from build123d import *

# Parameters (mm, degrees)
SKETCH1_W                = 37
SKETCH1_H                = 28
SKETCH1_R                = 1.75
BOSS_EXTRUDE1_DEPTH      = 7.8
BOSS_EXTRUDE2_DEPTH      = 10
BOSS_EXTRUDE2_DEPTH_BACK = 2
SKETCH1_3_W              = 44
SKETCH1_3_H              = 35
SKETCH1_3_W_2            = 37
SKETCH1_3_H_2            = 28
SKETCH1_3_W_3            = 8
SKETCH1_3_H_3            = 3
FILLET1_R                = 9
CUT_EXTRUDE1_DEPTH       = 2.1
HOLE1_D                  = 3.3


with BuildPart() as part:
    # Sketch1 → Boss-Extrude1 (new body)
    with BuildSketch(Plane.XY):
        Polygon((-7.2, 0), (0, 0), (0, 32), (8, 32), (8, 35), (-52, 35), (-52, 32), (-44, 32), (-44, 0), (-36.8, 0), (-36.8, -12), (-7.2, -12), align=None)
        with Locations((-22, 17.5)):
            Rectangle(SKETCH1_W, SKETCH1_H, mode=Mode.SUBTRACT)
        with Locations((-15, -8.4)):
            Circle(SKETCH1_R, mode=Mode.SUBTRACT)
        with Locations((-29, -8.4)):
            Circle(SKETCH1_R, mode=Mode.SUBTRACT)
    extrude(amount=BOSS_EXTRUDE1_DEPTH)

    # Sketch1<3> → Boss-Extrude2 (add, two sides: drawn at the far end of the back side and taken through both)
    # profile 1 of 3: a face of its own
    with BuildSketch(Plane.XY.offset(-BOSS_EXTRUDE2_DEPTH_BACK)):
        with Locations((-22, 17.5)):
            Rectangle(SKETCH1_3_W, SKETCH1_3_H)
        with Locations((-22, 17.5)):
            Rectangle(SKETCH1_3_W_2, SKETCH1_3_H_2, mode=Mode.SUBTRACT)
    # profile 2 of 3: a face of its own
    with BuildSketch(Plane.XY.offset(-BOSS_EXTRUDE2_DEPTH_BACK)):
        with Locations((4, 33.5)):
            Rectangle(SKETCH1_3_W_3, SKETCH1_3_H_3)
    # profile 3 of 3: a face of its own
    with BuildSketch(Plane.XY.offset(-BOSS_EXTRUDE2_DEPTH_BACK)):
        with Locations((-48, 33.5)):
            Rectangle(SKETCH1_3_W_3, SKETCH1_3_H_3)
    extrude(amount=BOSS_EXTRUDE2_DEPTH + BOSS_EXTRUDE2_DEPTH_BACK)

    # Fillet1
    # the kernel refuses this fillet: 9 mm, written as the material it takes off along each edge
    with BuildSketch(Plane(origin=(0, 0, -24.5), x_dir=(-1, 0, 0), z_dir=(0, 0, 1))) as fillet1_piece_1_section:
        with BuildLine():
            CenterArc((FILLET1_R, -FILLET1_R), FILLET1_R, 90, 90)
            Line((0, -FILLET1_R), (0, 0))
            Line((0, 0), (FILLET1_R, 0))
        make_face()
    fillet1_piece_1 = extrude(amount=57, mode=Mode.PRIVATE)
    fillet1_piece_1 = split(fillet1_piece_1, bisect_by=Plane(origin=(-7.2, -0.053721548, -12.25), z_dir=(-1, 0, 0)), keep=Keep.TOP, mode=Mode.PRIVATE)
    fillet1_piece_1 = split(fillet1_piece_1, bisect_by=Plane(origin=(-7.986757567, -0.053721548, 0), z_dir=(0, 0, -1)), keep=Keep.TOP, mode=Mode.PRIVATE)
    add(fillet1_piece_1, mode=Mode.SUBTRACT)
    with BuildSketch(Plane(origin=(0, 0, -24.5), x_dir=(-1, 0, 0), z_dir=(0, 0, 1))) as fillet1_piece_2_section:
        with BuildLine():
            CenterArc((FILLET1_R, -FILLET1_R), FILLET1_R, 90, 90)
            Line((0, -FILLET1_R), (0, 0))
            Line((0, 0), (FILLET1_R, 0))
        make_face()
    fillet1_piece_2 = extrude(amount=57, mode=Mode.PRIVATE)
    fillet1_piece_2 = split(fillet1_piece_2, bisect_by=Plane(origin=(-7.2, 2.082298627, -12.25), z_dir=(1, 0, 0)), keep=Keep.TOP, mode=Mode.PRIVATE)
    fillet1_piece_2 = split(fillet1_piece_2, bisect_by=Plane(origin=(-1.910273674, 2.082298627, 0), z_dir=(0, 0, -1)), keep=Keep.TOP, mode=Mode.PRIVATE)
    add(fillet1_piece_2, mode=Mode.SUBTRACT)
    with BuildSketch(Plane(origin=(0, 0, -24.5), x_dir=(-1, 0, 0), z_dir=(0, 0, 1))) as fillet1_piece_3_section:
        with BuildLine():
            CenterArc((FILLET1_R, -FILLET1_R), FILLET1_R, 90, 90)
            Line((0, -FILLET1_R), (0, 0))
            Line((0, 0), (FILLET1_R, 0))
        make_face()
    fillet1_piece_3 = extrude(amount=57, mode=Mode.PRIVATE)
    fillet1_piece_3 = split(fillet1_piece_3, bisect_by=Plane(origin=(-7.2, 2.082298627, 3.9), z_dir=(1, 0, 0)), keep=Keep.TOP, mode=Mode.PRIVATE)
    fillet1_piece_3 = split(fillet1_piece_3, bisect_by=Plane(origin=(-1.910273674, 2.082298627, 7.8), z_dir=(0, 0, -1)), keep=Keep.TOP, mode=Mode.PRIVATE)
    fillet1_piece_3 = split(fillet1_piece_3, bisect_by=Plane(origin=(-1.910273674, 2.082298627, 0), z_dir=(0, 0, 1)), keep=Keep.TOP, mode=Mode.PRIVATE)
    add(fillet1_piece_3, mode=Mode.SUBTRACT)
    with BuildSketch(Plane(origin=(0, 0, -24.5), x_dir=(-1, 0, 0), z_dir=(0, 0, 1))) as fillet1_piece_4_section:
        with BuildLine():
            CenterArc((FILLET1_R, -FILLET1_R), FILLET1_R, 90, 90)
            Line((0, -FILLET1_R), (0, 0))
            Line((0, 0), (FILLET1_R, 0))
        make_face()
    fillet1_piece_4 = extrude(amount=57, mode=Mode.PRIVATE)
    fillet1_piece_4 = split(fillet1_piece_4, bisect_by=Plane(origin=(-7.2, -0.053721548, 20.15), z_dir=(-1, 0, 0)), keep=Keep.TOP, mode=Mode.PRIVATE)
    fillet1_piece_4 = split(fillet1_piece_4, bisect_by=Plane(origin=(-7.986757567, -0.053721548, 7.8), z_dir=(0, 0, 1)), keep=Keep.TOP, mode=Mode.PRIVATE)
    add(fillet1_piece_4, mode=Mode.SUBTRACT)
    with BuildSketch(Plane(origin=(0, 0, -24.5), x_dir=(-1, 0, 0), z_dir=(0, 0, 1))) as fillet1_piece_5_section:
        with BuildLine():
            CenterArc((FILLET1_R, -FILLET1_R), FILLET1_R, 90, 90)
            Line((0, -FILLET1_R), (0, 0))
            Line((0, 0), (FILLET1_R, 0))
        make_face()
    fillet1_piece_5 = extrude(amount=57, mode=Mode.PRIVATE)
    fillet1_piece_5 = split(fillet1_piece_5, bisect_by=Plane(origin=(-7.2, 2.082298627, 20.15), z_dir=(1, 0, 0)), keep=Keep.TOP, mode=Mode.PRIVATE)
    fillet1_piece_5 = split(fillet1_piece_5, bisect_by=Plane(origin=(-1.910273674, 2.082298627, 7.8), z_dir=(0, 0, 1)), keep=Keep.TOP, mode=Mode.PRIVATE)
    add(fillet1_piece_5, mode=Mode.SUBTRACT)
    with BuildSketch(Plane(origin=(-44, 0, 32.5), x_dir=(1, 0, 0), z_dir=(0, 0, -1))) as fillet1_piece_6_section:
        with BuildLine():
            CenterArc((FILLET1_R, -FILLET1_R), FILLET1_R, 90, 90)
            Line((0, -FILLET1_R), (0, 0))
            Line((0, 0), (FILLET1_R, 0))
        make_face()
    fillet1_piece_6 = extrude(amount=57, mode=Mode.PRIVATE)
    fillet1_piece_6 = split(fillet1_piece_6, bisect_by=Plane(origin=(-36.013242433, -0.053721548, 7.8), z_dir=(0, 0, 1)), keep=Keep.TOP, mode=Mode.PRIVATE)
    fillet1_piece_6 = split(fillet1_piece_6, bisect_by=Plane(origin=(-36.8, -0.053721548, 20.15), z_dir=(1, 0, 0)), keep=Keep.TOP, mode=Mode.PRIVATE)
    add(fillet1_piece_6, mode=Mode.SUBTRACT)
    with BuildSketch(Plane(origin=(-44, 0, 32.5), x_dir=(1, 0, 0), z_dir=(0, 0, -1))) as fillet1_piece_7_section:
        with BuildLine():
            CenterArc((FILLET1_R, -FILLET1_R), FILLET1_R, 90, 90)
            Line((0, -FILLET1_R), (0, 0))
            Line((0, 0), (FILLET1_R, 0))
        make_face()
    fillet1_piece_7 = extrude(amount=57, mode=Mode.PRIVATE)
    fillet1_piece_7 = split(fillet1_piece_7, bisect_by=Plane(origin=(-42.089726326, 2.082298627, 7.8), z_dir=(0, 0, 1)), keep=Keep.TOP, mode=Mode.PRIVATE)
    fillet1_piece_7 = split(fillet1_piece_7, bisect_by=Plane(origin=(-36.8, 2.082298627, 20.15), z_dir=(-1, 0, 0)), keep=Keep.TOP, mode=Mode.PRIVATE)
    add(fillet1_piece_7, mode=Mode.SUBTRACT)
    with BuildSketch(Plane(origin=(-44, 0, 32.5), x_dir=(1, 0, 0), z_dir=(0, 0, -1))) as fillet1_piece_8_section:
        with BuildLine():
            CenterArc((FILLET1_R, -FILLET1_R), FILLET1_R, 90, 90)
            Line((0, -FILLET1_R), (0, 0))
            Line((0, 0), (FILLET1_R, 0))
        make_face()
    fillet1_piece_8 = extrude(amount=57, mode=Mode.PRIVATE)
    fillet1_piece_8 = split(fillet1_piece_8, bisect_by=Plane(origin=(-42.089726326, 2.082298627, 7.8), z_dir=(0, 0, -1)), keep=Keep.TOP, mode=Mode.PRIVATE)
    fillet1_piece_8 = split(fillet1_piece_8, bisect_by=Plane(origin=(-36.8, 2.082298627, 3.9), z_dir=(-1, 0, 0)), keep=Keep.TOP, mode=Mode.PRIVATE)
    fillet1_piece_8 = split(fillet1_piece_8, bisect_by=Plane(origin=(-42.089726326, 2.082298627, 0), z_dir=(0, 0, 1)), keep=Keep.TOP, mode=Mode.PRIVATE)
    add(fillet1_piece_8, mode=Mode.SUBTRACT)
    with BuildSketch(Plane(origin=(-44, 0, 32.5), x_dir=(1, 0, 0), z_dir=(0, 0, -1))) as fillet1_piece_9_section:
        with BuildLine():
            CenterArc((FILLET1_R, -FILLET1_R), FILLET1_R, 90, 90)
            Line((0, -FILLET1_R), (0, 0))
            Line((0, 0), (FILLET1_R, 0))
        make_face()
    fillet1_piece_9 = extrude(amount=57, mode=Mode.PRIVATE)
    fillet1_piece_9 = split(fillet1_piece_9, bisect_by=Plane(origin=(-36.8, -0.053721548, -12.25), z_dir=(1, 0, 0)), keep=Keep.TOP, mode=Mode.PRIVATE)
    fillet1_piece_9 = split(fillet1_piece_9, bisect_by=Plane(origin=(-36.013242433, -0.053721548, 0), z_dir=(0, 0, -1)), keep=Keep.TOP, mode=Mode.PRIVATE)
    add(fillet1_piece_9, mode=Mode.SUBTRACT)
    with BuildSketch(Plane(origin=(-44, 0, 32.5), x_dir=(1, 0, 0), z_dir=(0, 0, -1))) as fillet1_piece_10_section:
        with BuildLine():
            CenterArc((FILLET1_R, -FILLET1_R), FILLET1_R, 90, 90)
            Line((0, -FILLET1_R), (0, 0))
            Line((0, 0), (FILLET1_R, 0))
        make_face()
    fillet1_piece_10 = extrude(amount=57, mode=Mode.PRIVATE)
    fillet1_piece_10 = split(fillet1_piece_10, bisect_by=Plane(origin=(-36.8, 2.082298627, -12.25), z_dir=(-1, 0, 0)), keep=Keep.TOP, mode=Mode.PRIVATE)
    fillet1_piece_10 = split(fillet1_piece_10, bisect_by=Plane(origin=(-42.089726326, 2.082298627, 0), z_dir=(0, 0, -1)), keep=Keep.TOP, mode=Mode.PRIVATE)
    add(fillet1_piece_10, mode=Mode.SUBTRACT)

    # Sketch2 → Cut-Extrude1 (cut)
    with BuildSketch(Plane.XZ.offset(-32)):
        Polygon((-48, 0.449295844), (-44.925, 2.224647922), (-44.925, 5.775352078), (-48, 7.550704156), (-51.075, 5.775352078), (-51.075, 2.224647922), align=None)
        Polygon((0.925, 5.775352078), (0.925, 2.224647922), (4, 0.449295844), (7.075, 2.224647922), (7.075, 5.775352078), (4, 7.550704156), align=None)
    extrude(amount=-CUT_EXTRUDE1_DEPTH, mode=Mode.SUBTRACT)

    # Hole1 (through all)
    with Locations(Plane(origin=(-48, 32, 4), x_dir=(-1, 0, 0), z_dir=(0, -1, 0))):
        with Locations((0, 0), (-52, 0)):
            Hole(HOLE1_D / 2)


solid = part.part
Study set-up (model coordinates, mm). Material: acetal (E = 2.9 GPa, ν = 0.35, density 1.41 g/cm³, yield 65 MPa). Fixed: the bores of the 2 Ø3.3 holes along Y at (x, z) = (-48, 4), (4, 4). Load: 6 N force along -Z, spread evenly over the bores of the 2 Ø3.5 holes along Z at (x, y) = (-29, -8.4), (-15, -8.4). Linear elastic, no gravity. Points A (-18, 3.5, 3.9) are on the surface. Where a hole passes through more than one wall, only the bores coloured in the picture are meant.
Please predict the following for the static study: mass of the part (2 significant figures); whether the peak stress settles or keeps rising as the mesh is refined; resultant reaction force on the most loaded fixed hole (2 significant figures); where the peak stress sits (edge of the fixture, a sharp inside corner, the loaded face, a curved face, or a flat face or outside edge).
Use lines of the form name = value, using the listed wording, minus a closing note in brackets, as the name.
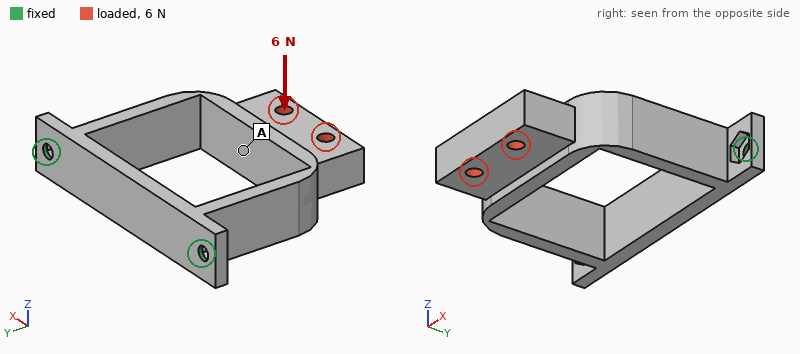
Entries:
mass of the part = 12 g
whether the peak stress settles or keeps rising as the mesh is refined = keeps rising
resultant reaction force on the most loaded fixed hole = 3.0 N
where the peak stress sits = edge of the fixture
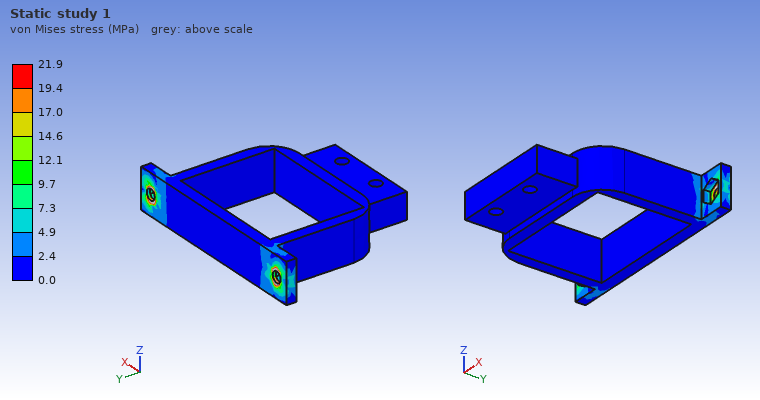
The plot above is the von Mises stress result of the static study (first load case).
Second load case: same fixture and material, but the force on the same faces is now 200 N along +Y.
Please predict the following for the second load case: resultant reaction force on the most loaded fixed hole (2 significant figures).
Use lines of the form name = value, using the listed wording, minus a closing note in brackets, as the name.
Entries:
resultant reaction force on the most loaded fixed hole = 120 N
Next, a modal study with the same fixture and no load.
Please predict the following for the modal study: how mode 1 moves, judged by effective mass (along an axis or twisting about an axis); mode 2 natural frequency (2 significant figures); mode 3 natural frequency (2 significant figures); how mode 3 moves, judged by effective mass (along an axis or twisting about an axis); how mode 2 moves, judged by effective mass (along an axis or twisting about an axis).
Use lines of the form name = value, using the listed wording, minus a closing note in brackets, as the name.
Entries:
how mode 1 moves, judged by effective mass = along Z
mode 2 natural frequency = 380 Hz
mode 3 natural frequency = 980 Hz
how mode 3 moves, judged by effective mass = twisting about Y
how mode 2 moves, judged by effective mass = along X
